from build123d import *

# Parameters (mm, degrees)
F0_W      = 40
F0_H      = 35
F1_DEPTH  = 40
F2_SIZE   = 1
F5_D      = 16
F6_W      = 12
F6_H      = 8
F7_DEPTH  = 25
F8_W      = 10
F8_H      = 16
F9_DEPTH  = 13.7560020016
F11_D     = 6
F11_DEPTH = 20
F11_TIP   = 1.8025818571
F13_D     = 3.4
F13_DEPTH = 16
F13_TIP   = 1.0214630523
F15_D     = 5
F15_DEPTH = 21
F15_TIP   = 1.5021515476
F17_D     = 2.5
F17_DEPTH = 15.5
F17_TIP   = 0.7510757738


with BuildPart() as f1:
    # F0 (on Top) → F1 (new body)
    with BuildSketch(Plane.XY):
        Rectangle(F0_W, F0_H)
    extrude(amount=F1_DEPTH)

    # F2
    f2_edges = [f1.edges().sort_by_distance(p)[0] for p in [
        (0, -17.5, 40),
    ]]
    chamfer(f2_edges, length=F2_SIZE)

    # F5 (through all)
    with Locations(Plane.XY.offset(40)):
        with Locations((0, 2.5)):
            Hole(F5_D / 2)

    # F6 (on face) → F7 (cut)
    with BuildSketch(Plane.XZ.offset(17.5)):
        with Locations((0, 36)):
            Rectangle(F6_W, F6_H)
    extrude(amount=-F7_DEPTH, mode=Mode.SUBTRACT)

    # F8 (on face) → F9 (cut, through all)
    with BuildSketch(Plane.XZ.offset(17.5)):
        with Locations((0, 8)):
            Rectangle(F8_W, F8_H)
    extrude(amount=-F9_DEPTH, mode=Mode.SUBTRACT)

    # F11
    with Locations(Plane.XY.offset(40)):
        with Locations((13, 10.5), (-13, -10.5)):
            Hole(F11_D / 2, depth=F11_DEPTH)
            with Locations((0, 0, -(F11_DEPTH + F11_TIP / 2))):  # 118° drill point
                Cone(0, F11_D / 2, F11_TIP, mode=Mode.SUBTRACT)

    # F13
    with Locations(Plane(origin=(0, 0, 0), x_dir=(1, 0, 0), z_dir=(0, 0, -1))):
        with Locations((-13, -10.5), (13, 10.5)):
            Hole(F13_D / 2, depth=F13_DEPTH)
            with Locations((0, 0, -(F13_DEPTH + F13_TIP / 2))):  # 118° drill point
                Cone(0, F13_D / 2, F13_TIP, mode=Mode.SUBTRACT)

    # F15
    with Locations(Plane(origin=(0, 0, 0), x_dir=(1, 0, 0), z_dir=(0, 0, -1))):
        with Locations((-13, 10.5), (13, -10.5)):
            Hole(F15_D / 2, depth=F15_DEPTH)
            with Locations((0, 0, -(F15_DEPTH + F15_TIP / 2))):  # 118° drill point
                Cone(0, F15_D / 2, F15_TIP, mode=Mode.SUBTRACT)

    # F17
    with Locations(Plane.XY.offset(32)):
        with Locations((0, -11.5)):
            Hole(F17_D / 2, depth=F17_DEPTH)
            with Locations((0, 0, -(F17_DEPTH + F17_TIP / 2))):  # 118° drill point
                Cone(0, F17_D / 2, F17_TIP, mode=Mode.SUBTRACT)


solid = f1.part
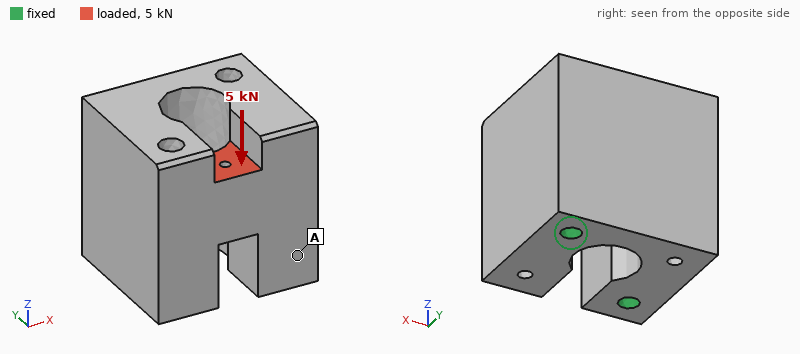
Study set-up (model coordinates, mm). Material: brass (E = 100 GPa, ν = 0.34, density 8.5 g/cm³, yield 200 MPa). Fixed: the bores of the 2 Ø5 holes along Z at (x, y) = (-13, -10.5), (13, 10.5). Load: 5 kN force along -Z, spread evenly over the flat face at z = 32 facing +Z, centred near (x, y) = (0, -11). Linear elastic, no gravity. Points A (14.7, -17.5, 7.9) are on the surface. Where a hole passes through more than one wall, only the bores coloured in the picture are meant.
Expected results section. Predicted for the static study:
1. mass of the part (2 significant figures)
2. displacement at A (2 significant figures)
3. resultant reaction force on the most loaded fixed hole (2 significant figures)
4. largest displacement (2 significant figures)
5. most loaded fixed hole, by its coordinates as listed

360 g
7.8 µm
3.3 kN
12 µm
(-13, -10.5)
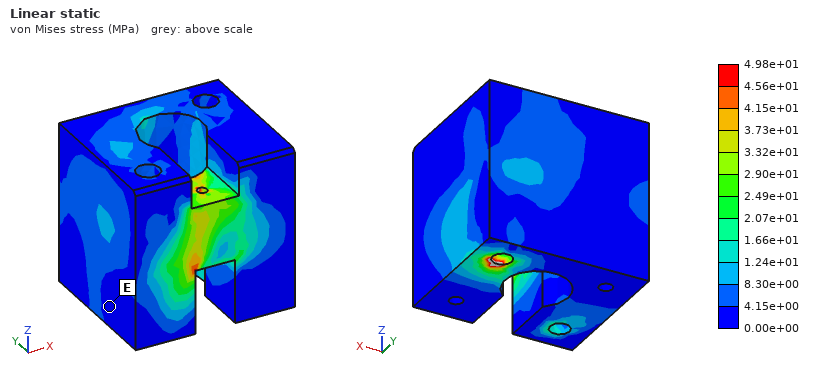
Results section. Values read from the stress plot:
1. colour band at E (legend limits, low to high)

0.00e+00 to 4.15e+00 MPa
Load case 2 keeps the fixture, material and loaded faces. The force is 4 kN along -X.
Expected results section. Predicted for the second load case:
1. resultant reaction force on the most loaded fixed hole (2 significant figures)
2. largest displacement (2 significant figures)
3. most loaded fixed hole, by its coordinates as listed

3.4 kN
12 µm
(-13, -10.5)
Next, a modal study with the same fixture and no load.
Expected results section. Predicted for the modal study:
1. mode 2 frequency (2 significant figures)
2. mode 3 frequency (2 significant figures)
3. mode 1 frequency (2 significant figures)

11 kHz
13 kHz
6700 Hz
